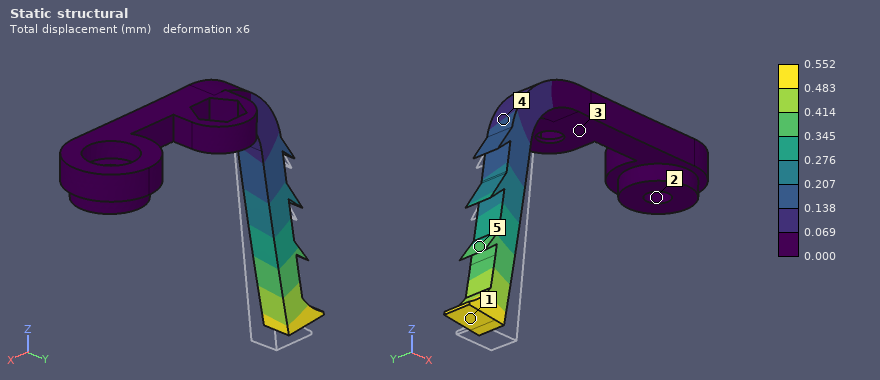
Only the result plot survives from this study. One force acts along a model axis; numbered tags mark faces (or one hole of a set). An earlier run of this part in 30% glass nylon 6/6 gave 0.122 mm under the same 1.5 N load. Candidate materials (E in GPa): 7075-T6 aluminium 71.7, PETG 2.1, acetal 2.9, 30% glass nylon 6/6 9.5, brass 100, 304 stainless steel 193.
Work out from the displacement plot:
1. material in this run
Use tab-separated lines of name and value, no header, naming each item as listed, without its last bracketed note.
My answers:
material in this run	PETG
